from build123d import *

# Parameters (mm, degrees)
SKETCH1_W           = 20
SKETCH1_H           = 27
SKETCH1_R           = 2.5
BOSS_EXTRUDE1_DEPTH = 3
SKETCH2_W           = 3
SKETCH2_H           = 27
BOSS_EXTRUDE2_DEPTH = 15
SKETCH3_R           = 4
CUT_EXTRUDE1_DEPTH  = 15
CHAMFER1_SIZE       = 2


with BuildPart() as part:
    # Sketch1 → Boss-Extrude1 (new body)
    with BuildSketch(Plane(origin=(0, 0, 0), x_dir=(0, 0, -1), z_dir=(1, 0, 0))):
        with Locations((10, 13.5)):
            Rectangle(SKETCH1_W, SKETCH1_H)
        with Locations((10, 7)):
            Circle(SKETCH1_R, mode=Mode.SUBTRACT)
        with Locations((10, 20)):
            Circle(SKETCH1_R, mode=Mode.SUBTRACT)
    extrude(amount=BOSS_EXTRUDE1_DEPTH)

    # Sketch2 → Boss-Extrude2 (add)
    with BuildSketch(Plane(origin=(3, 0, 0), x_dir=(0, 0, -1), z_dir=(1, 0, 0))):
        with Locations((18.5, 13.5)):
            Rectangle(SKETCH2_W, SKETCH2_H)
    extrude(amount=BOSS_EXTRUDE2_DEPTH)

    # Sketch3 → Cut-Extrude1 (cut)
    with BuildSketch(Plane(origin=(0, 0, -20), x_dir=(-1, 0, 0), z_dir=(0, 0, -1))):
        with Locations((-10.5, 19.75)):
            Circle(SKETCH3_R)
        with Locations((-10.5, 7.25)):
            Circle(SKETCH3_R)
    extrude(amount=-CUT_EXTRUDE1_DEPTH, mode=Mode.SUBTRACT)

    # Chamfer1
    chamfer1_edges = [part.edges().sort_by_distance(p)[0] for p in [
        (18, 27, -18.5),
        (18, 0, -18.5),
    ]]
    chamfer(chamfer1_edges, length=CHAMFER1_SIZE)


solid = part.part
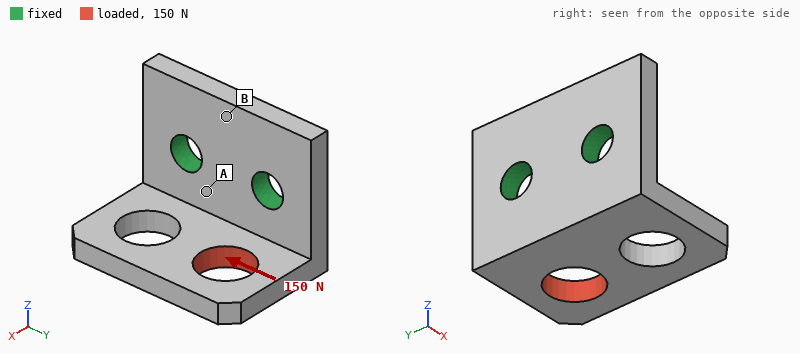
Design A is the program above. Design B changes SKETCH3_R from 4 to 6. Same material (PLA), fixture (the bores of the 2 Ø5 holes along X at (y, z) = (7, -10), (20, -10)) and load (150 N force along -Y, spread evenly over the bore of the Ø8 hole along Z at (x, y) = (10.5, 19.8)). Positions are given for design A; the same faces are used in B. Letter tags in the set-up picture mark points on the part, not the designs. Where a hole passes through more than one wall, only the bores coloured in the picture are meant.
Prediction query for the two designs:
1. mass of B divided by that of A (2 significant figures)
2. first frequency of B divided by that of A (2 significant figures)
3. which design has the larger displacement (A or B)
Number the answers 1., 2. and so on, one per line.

1. 0.84
2. 0.94
3. B
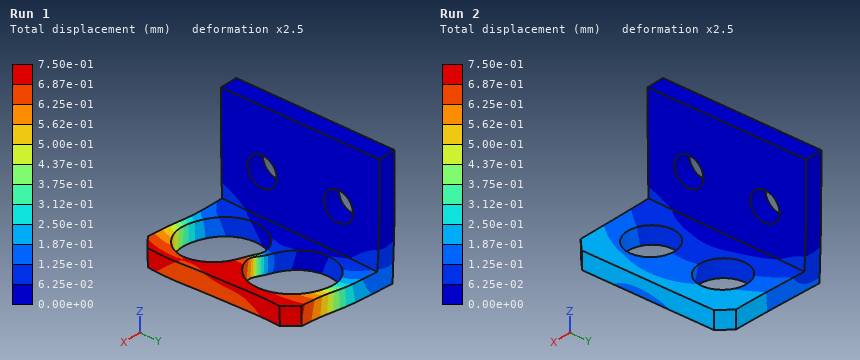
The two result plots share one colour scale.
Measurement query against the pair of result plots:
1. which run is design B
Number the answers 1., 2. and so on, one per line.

1. Run 1
